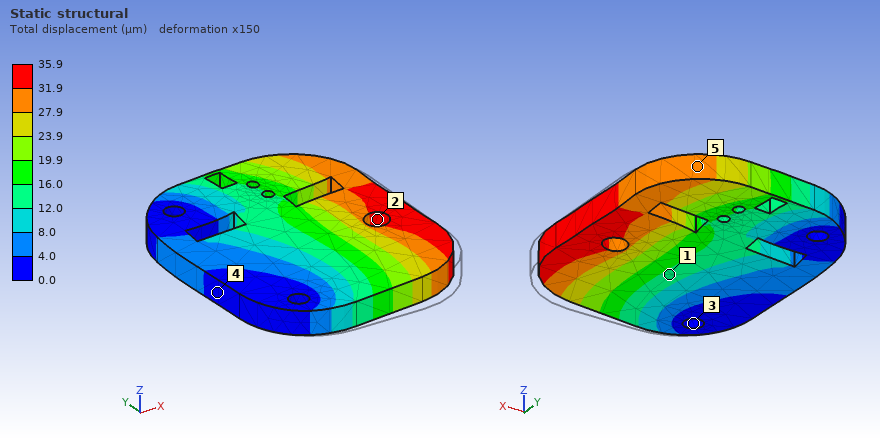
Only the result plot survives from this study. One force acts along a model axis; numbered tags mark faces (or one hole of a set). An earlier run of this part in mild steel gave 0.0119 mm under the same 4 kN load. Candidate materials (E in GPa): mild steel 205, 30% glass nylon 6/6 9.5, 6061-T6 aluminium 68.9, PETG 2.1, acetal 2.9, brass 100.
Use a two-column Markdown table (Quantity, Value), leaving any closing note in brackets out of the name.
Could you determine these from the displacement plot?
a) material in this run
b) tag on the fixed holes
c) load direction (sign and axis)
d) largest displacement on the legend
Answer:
| Quantity | Value |
|---|---|
| material in this run | 6061-T6 aluminium |
| tag on the fixed holes | 3 |
| load direction | +Y |
| largest displacement on the legend | 35.9 µm |
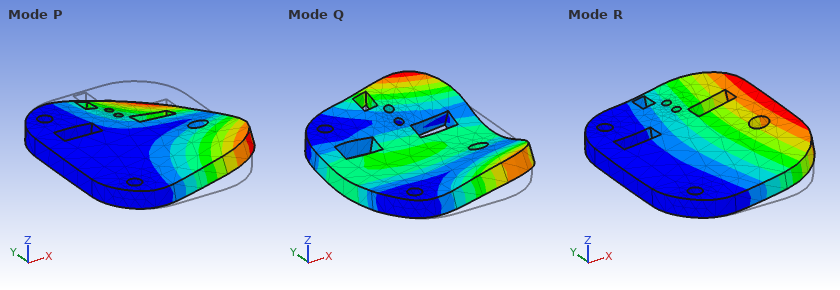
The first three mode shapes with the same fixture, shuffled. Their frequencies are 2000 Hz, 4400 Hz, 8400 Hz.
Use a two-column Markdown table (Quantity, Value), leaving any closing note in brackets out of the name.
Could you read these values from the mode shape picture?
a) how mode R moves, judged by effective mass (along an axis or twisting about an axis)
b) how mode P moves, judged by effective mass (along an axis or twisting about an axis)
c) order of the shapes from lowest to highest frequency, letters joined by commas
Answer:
| Quantity | Value |
|---|---|
| how mode R moves, judged by effective mass | along Z |
| how mode P moves, judged by effective mass | twisting about X |
| order of the shapes from lowest to highest frequency, letters joined by commas | R, P, Q |
